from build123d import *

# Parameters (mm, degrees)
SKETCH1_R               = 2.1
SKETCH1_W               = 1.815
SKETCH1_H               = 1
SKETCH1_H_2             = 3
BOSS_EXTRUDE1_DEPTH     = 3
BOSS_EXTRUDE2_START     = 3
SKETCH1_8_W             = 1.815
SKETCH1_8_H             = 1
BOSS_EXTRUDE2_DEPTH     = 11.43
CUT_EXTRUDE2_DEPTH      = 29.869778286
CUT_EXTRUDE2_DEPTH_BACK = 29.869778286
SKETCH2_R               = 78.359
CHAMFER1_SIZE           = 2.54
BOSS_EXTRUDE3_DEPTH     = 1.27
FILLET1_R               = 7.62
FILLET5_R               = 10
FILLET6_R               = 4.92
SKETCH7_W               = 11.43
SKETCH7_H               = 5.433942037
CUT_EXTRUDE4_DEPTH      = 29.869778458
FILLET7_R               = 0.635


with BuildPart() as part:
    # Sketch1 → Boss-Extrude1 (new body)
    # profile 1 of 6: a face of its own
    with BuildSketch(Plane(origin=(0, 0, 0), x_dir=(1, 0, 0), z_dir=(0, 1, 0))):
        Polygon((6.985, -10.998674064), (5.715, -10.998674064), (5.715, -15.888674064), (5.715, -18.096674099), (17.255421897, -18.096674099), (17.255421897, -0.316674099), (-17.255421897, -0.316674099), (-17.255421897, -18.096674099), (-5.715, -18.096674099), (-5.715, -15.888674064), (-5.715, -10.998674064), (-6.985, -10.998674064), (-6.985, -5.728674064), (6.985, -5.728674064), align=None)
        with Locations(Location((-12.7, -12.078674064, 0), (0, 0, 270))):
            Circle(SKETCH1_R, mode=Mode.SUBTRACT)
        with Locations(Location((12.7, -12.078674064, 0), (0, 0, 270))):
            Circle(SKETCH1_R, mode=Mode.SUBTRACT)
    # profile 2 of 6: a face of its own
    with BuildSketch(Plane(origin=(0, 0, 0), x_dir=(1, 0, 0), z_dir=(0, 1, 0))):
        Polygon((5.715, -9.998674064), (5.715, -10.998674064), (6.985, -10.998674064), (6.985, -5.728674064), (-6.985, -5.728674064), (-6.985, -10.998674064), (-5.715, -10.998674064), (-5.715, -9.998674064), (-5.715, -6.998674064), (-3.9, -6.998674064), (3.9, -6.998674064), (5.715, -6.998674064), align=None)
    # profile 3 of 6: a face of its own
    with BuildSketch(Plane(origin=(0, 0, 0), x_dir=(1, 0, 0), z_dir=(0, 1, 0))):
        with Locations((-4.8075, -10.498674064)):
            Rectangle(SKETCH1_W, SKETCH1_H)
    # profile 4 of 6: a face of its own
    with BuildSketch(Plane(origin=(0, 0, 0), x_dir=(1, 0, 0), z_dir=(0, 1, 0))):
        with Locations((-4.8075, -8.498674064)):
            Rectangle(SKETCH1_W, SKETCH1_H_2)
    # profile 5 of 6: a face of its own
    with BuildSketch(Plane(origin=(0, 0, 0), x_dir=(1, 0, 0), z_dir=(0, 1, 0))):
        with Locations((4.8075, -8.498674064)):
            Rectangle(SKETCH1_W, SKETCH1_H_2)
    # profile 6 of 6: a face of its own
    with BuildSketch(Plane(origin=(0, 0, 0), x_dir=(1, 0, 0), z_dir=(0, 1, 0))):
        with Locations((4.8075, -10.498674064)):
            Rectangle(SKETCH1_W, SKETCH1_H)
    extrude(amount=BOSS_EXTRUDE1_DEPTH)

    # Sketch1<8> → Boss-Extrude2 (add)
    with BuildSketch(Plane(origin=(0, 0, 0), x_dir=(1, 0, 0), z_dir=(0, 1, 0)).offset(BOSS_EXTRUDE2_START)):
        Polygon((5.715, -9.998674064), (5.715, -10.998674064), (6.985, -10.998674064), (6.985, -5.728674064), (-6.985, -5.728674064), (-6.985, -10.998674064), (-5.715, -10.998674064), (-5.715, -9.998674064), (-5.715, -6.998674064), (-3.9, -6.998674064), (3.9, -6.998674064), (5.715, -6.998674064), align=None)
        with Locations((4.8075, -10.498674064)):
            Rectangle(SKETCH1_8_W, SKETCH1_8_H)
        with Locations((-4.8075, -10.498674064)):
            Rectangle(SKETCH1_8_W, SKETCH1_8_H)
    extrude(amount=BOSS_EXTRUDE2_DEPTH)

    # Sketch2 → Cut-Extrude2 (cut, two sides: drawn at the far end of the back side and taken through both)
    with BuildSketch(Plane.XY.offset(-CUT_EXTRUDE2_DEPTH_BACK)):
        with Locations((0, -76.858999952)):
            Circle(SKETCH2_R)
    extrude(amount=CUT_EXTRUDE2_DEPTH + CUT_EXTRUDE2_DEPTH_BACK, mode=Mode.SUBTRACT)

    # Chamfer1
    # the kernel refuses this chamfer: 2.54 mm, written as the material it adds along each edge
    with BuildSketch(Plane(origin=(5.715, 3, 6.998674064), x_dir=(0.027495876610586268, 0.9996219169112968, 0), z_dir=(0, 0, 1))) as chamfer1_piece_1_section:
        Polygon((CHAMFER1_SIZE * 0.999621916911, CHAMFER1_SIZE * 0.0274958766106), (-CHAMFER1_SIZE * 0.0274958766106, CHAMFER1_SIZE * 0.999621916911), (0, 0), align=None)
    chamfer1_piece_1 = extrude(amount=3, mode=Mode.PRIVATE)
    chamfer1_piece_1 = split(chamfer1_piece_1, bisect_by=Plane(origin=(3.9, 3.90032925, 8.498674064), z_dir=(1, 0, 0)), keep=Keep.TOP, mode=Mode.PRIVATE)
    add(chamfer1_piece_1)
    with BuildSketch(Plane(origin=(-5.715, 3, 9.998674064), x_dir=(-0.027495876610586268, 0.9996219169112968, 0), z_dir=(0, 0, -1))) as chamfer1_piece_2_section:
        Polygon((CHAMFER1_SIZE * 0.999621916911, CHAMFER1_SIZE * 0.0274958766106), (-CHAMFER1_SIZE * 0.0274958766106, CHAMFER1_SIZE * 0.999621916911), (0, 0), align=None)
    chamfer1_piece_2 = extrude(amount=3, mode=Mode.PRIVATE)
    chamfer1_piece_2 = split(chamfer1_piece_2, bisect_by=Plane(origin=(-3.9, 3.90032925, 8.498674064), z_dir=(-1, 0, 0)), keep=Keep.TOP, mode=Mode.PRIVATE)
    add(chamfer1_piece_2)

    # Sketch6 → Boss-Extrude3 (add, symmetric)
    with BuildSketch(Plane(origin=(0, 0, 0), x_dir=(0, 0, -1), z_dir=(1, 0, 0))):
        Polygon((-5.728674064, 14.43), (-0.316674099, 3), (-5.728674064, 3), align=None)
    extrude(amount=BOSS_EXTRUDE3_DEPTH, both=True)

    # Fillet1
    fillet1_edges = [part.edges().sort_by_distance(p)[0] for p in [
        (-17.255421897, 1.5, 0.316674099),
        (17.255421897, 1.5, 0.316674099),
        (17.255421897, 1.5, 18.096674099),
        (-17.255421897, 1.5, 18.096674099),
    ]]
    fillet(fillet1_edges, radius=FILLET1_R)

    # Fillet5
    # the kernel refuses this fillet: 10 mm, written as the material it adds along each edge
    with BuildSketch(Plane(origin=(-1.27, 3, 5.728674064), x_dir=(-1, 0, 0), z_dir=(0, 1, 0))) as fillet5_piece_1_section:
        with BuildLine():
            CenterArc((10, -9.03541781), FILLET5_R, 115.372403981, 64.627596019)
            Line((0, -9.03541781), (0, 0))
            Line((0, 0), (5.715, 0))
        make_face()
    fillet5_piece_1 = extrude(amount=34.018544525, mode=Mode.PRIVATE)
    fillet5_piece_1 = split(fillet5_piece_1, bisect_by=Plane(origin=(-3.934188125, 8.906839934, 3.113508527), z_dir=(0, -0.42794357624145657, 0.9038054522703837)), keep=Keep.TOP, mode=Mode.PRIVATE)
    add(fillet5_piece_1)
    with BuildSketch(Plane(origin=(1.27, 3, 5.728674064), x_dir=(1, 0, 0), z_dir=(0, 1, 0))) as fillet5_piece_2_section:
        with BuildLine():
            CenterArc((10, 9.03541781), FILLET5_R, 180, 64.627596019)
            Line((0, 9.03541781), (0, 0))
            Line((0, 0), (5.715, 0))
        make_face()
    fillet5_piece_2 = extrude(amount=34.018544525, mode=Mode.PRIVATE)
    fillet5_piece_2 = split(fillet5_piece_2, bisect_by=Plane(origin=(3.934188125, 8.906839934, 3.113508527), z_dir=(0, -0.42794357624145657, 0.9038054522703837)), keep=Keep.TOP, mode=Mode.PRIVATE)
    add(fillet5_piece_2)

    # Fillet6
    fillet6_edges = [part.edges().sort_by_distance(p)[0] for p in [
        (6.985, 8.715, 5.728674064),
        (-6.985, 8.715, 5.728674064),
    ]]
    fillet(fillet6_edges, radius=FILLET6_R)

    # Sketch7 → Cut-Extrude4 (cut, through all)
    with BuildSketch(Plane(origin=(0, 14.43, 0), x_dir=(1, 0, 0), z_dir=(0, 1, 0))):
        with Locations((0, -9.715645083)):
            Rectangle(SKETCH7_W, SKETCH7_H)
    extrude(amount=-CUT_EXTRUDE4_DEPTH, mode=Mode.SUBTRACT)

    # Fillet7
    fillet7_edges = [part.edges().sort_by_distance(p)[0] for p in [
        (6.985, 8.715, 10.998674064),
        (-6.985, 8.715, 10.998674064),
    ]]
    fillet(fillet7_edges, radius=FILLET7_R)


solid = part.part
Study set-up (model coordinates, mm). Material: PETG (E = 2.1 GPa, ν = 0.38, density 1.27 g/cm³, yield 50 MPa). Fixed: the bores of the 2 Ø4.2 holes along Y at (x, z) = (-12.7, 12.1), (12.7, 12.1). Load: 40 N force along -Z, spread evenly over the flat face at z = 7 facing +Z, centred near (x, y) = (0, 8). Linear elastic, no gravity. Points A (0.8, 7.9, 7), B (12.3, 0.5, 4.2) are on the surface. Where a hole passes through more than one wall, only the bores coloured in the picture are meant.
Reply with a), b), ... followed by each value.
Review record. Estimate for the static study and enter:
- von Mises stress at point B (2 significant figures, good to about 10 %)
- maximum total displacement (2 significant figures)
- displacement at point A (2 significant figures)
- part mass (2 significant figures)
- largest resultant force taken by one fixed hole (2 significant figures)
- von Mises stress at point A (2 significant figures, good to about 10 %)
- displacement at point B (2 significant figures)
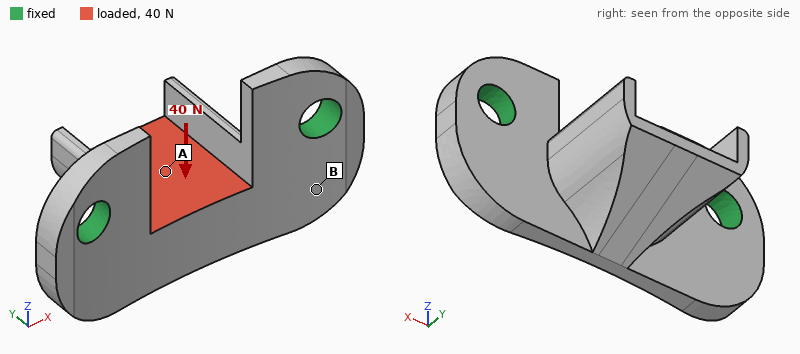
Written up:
a) 5.7 MPa
b) 0.42 mm
c) 0.20 mm
d) 1.9 g
e) 20 N
f) 2.4 MPa
g) 0.065 mm
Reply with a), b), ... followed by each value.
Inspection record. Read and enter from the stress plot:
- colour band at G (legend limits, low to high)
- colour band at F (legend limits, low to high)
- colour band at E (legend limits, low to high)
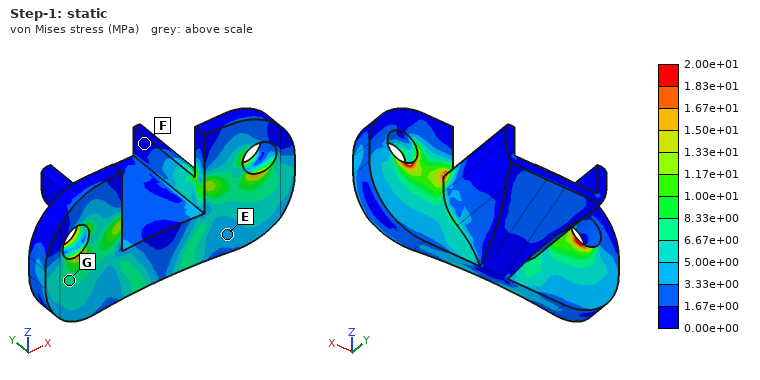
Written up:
a) 6.67e+00 to 8.33e+00 MPa
b) 0.00e+00 to 1.67e+00 MPa
c) 3.33e+00 to 5.00e+00 MPa
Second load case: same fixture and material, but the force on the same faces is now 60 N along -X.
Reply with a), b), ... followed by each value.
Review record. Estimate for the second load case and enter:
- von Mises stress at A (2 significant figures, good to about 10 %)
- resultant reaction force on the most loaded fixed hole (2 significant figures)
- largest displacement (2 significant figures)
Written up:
a) 4.5 MPa
b) 36 N
c) 0.17 mm
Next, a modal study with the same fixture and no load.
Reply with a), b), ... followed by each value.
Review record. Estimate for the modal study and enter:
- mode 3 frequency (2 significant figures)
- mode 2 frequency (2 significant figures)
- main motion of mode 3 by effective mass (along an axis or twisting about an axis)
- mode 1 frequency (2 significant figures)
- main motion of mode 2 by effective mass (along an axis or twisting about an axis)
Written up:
a) 5100 Hz
b) 4300 Hz
c) along Y
d) 1800 Hz
e) along X
